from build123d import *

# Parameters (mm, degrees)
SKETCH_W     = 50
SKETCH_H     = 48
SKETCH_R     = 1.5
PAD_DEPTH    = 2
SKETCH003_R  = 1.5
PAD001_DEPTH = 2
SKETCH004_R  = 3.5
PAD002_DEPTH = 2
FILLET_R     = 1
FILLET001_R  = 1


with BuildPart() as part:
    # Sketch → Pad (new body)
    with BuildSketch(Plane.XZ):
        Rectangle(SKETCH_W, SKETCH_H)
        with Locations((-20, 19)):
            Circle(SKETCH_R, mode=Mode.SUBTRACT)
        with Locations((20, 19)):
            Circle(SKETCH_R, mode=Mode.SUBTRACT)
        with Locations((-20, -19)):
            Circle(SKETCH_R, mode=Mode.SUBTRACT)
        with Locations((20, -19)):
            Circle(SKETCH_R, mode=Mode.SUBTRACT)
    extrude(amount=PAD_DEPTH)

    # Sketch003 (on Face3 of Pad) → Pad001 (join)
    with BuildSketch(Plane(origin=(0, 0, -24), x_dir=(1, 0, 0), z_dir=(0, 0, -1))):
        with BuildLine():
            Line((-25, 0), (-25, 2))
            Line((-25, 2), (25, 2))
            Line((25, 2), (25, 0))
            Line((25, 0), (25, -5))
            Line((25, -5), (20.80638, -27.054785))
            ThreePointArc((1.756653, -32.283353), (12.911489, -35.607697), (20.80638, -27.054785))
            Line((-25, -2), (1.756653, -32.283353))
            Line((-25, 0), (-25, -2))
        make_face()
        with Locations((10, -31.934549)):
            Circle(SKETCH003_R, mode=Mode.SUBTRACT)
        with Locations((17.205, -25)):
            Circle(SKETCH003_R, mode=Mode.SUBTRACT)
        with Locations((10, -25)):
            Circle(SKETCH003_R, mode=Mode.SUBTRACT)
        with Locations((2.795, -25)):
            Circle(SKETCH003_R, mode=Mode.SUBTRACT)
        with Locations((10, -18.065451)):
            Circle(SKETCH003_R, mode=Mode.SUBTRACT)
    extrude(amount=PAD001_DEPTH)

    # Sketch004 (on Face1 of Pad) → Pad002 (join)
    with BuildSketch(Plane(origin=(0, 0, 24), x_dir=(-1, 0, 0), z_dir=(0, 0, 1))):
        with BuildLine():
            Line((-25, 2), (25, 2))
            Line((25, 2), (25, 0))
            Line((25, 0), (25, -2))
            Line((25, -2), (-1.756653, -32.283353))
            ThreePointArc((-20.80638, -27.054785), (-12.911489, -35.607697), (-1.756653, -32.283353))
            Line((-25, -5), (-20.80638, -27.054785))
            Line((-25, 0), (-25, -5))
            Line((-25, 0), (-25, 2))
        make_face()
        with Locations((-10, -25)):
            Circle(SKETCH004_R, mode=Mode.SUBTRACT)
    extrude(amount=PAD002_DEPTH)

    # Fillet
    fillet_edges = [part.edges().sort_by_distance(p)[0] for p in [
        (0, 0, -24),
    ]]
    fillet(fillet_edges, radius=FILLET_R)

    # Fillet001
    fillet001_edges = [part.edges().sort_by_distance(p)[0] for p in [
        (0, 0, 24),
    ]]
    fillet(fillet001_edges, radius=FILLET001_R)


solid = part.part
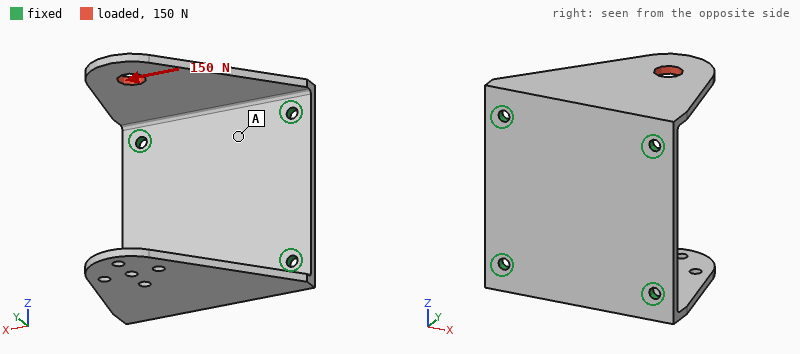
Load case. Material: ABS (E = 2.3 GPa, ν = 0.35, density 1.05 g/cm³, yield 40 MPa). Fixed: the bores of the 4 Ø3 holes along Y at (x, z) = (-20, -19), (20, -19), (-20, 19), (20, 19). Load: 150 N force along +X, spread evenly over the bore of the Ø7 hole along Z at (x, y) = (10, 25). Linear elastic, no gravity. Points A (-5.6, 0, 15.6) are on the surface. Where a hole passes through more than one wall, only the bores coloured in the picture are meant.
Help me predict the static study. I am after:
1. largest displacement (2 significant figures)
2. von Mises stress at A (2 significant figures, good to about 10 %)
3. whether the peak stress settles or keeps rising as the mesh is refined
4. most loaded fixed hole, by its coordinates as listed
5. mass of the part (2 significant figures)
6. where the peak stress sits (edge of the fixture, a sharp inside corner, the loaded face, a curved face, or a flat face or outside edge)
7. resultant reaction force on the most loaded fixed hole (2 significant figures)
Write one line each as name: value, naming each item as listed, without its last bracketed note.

largest displacement: 0.89 mm
von Mises stress at A: 3.5 MPa
whether the peak stress settles or keeps rising as the mesh is refined: keeps rising
most loaded fixed hole, by its coordinates as listed: (-20, 19)
mass of the part: 10 g
where the peak stress sits: edge of the fixture
resultant reaction force on the most loaded fixed hole: 130 N
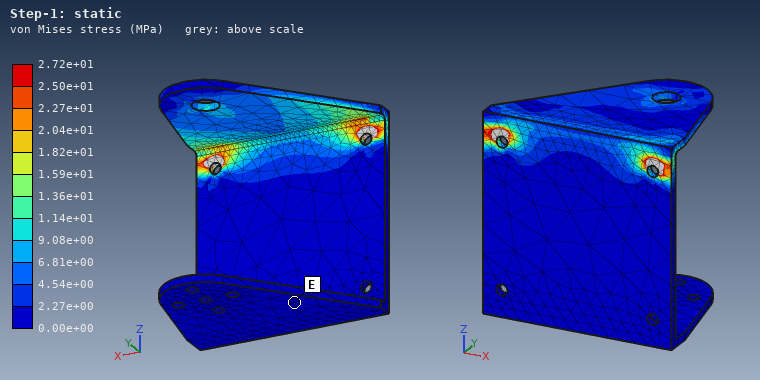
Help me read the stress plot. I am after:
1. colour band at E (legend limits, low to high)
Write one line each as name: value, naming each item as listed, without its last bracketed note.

colour band at E: 0.00e+00 to 2.27e+00 MPa
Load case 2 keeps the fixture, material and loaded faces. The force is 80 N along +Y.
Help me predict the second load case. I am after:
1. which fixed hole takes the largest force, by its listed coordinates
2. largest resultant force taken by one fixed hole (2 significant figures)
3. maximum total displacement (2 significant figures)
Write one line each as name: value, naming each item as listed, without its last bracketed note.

which fixed hole takes the largest force, by its listed coordinates: (20, 19)
largest resultant force taken by one fixed hole: 62 N
maximum total displacement: 0.89 mm
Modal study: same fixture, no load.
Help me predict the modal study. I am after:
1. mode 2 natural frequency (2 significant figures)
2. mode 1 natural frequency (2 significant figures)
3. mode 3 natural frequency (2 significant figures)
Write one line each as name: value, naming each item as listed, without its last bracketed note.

mode 2 natural frequency: 420 Hz
mode 1 natural frequency: 410 Hz
mode 3 natural frequency: 1300 Hz
